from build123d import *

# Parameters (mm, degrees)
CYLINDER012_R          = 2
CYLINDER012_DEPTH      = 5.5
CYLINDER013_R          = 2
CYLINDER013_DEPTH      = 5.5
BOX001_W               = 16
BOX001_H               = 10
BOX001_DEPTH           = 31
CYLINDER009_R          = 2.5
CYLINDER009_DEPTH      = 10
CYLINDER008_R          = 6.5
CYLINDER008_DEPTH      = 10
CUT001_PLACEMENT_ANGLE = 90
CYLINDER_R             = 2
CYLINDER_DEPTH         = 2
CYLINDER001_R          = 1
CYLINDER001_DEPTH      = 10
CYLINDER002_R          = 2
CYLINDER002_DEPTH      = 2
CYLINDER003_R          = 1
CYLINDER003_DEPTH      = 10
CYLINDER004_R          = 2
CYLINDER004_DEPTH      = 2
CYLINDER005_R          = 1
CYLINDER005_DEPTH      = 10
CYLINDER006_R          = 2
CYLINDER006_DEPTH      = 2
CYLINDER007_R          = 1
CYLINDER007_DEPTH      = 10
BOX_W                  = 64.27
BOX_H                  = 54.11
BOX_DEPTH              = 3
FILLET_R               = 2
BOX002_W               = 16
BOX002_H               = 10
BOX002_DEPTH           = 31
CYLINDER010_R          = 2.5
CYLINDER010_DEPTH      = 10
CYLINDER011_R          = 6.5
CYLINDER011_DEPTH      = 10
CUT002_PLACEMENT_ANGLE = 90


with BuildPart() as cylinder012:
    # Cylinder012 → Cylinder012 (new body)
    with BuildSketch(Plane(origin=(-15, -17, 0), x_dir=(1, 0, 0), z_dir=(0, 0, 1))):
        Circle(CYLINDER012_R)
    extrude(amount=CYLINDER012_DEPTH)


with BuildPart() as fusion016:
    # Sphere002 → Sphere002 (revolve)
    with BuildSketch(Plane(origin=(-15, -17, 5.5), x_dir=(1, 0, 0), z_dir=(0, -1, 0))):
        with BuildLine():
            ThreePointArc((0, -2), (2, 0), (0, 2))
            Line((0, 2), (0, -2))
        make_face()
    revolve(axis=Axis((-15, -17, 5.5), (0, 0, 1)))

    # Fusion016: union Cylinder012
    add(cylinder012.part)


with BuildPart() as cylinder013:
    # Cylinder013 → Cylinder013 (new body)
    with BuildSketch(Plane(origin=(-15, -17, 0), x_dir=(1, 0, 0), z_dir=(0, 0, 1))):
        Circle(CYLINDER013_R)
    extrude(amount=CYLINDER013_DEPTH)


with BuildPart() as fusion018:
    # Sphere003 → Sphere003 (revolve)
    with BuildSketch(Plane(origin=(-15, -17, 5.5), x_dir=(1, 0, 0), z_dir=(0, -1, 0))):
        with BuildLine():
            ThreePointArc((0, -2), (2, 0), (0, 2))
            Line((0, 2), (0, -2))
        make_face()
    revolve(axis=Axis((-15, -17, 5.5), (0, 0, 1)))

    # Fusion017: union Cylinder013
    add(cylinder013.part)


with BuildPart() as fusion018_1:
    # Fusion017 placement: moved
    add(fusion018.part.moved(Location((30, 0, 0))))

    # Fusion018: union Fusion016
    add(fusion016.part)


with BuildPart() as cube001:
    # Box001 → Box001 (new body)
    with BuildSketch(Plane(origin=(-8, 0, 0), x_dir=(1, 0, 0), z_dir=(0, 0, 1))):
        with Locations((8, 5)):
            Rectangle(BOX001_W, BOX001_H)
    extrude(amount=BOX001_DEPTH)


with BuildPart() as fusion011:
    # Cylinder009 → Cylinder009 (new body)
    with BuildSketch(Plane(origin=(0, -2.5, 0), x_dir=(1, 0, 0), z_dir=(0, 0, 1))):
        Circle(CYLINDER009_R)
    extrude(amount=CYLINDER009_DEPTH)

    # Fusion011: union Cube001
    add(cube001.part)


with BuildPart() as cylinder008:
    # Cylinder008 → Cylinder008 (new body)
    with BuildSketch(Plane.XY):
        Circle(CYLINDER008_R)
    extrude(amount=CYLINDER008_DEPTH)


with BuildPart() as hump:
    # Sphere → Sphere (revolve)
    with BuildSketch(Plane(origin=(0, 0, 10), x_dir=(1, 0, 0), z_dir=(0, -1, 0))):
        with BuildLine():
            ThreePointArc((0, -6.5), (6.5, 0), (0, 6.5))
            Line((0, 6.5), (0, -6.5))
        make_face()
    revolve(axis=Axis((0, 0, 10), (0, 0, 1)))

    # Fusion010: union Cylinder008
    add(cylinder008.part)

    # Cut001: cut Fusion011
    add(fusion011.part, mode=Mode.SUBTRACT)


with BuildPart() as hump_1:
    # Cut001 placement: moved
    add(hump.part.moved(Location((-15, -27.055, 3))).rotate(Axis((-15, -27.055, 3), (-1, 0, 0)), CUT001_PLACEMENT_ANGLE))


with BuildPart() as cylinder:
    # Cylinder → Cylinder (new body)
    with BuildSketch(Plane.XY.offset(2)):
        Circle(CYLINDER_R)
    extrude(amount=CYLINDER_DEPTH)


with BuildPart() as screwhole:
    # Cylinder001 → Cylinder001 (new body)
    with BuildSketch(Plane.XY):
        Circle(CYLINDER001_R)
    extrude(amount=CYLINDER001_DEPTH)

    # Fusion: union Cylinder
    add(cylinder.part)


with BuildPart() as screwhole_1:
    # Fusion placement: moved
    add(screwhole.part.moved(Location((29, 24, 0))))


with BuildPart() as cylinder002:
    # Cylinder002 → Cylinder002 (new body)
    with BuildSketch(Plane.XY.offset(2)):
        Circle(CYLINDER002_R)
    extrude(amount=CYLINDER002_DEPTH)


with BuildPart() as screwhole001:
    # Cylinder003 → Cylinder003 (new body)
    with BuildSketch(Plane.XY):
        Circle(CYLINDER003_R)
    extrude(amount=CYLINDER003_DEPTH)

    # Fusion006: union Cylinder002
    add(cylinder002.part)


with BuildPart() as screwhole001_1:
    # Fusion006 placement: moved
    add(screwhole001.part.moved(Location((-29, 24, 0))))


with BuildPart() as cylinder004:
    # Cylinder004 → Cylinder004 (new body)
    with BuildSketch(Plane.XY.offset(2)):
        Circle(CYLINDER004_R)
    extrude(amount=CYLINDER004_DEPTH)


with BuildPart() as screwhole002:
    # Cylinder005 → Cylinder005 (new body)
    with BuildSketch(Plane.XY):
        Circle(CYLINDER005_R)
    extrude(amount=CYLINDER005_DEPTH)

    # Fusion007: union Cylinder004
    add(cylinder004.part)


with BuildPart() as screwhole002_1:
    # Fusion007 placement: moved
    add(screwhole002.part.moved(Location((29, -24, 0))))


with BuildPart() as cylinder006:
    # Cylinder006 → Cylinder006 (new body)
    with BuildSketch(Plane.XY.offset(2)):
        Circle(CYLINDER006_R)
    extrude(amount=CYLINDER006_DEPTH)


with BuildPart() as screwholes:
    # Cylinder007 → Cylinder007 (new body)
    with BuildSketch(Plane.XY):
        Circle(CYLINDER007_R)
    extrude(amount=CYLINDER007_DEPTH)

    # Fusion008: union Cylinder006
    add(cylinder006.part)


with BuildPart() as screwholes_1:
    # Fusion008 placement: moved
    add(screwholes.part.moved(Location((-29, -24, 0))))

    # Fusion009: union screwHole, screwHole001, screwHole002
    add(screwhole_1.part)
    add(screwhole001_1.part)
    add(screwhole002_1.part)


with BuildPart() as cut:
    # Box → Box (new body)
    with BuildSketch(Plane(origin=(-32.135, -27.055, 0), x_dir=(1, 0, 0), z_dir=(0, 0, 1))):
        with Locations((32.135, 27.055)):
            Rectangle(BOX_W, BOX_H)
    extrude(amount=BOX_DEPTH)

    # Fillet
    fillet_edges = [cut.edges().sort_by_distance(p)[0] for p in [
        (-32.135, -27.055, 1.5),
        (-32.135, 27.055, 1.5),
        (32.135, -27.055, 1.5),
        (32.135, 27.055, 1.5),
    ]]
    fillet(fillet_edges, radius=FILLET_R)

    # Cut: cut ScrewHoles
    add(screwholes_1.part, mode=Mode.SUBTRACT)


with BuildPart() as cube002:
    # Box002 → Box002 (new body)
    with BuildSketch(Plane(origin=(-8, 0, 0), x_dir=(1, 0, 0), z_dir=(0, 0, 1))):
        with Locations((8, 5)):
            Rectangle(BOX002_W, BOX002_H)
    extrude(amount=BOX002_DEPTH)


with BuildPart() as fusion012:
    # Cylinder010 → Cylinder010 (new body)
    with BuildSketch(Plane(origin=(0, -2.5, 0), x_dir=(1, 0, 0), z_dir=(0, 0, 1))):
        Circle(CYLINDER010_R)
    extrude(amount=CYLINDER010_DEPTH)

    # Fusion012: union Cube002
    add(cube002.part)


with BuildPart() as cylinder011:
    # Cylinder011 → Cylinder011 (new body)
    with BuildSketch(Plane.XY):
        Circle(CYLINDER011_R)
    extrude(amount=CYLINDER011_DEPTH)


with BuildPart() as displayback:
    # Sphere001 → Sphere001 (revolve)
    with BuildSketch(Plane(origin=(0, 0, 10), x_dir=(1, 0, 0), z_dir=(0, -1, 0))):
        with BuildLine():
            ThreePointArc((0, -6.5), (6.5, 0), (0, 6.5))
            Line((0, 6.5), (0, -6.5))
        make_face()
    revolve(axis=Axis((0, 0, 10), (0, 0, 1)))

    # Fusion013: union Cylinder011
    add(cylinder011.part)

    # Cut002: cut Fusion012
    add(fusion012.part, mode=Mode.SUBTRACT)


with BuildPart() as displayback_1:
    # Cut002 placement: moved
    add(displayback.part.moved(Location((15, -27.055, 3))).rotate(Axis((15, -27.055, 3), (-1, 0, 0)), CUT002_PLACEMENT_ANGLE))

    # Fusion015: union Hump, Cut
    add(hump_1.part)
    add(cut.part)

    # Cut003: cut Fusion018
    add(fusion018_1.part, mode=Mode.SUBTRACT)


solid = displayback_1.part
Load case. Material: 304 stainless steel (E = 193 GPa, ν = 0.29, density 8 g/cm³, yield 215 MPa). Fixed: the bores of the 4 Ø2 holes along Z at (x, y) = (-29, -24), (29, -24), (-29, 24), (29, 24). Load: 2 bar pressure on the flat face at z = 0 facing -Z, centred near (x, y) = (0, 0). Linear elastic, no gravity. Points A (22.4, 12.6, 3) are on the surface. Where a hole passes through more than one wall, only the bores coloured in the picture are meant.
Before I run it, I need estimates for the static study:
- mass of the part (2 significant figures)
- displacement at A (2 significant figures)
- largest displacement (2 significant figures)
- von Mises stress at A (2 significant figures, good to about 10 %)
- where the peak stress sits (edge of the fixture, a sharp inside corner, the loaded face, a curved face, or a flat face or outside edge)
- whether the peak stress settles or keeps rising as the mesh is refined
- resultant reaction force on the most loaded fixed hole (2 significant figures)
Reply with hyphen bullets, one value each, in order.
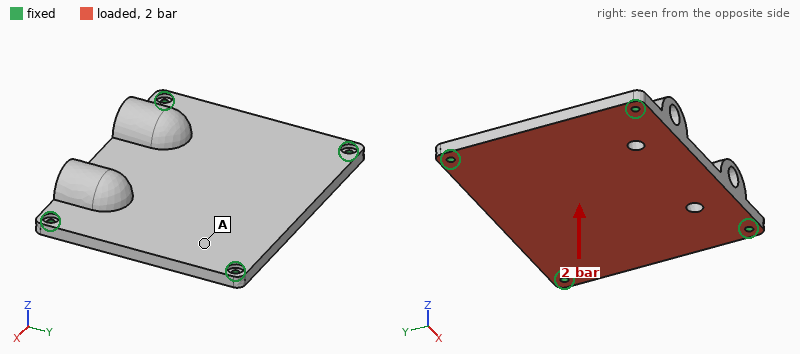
- 94 g
- 17 µm
- 38 µm
- 16 MPa
- edge of the fixture
- keeps rising
- 250 N
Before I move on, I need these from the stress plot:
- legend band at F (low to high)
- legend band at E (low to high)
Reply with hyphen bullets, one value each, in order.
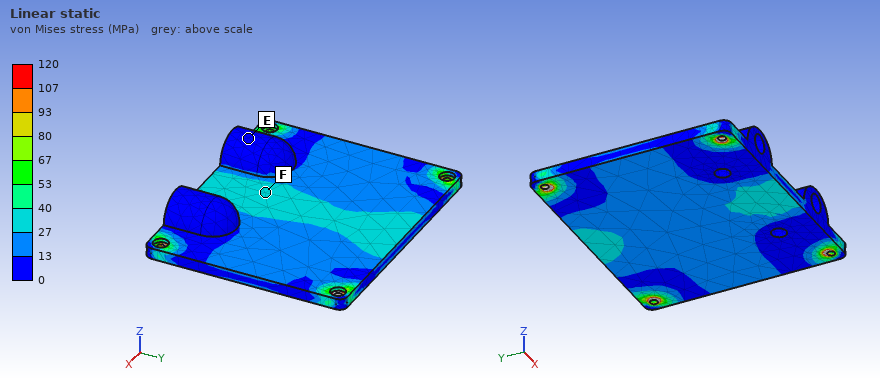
- 27 to 40 MPa
- 0 to 13 MPa
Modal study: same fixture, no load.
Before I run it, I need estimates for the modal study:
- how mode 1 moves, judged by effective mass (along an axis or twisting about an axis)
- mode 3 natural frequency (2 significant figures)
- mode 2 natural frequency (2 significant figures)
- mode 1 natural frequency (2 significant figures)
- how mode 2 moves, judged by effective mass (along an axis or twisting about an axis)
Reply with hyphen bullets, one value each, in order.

- along Z
- 5800 Hz
- 4700 Hz
- 2600 Hz
- twisting about X
